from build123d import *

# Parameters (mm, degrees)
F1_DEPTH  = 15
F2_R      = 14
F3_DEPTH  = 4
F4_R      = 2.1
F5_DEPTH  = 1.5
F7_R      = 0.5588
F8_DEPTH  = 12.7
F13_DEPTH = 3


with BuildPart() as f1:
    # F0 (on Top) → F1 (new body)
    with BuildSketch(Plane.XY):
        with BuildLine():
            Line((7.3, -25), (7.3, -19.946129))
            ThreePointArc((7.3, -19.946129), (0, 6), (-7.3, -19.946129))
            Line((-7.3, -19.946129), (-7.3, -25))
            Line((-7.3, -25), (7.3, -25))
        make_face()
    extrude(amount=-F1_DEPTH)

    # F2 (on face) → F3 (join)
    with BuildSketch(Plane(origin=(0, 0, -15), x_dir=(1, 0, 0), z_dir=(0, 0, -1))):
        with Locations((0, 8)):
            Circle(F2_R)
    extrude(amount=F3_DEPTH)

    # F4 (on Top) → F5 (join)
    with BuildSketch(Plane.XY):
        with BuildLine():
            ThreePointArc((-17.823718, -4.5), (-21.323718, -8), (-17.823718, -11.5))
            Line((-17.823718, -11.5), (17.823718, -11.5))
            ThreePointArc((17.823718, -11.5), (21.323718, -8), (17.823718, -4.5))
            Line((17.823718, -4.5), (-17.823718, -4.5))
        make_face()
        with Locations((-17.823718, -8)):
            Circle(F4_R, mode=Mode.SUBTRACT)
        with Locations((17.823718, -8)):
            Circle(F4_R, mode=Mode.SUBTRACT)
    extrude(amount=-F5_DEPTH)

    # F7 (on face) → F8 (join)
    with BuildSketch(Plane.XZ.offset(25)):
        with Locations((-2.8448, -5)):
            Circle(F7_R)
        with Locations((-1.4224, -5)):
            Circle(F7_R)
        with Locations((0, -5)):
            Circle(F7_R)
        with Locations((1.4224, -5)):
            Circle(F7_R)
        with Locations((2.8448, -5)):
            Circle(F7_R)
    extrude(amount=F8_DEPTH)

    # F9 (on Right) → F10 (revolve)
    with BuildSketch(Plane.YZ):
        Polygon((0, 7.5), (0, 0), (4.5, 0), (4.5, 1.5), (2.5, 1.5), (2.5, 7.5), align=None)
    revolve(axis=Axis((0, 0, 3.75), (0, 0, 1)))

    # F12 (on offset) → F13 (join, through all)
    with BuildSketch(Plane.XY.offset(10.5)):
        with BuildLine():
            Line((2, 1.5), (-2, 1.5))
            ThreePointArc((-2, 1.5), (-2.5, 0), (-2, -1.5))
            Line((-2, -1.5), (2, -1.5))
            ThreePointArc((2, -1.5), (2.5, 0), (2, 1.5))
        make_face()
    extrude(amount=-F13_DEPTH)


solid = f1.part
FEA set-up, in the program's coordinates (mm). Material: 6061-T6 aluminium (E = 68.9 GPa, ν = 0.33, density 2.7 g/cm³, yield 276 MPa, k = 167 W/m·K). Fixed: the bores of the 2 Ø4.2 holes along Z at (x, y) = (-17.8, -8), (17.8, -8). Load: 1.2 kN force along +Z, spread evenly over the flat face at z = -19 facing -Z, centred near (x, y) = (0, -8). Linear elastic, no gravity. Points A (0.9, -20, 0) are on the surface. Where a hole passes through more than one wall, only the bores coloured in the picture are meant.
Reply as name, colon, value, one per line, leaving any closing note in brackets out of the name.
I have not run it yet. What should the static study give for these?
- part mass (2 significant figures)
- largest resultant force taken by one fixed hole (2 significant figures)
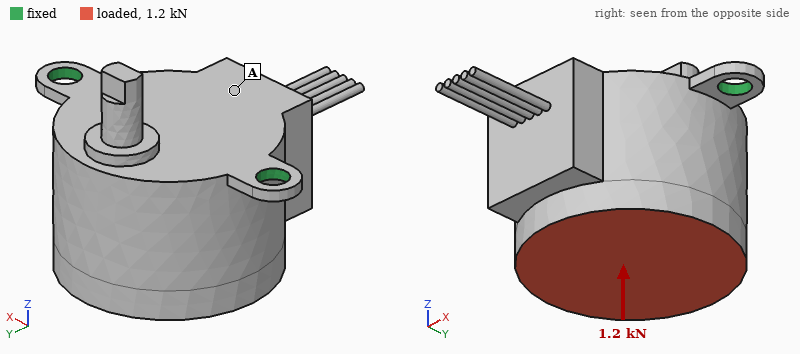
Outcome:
part mass: 35 g
largest resultant force taken by one fixed hole: 690 N
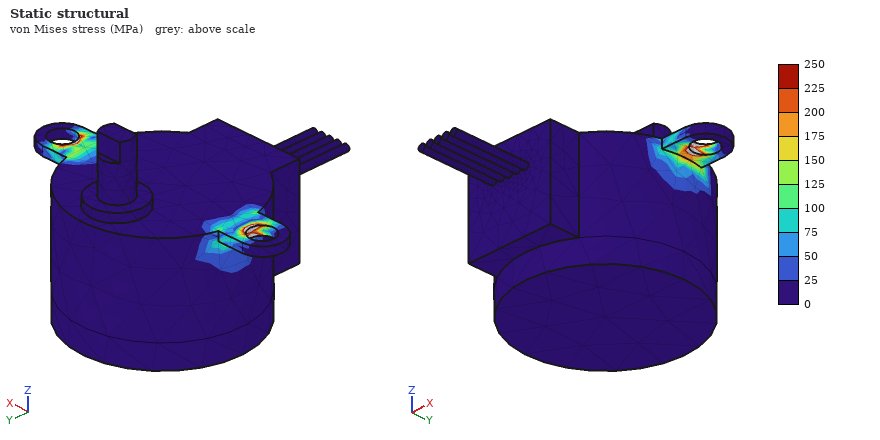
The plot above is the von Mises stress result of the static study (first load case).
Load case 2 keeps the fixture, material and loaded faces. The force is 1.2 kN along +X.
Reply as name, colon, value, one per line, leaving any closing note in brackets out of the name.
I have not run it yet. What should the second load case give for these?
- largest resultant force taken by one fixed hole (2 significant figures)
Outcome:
largest resultant force taken by one fixed hole: 950 N
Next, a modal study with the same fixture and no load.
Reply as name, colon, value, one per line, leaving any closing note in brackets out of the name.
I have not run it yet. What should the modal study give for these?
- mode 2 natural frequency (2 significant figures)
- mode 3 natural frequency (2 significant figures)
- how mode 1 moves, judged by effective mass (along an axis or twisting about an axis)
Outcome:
mode 2 natural frequency: 4700 Hz
mode 3 natural frequency: 4700 Hz
how mode 1 moves, judged by effective mass: along Y
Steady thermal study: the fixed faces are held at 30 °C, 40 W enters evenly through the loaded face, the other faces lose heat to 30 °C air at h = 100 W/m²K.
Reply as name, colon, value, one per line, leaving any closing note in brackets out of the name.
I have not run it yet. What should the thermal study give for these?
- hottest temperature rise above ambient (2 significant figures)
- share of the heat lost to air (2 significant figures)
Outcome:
hottest temperature rise above ambient: 41 K
share of the heat lost to air: 26 %
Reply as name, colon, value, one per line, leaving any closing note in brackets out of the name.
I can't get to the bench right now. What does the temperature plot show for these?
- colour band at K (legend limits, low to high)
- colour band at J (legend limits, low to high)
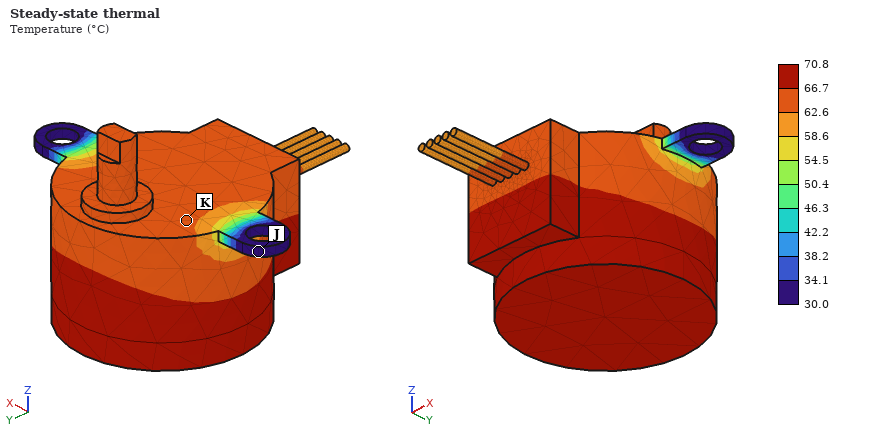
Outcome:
colour band at K: 62.6 to 66.7 °C
colour band at J: 30.0 to 34.1 °C
